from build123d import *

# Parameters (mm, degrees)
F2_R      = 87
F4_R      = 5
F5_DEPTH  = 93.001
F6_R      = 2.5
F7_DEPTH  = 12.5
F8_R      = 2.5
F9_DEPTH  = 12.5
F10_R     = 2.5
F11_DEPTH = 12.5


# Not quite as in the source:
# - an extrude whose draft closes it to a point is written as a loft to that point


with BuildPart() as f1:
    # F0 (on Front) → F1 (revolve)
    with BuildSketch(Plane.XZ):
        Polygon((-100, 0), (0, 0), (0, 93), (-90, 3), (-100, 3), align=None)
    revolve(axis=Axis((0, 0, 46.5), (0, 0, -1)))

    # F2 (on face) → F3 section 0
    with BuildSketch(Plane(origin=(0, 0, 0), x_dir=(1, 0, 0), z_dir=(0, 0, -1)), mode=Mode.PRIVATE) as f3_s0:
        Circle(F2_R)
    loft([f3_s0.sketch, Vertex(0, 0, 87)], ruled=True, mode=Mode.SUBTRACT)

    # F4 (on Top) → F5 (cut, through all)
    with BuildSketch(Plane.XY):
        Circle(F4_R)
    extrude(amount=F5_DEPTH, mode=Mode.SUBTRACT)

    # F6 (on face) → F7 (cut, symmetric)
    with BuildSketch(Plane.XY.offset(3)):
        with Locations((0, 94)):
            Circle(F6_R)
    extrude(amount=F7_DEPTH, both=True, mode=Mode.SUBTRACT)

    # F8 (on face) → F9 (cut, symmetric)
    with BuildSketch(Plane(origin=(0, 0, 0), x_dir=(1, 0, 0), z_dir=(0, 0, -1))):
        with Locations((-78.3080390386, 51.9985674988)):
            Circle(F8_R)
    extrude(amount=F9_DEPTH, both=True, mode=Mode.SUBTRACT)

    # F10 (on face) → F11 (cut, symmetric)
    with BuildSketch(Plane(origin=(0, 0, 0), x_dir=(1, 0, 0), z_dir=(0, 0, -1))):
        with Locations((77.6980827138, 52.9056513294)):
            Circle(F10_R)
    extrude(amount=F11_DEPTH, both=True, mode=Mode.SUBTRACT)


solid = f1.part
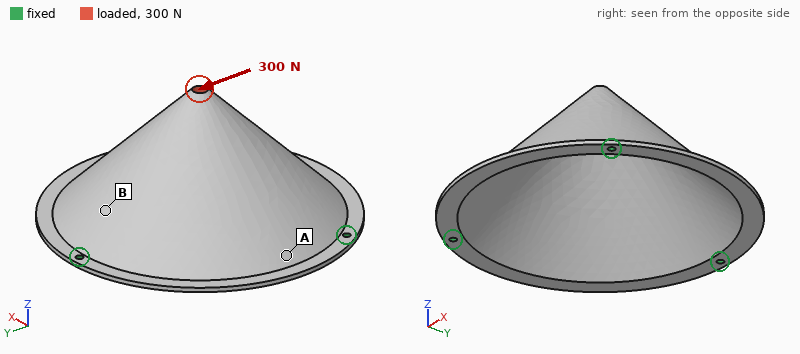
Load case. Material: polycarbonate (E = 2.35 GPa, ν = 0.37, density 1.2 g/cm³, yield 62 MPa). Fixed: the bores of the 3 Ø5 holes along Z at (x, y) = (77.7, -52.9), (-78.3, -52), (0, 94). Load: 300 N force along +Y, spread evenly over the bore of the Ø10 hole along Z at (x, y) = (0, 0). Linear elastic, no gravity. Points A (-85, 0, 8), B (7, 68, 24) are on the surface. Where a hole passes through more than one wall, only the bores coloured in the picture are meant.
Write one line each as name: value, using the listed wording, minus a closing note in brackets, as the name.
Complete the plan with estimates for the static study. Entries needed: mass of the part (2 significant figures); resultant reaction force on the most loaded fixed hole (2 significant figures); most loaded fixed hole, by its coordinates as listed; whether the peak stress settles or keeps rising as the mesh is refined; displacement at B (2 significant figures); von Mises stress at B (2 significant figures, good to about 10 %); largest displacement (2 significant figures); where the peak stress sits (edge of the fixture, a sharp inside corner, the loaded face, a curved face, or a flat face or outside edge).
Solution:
mass of the part: 200 g
resultant reaction force on the most loaded fixed hole: 260 N
most loaded fixed hole, by its coordinates as listed: (0, 94)
whether the peak stress settles or keeps rising as the mesh is refined: keeps rising
displacement at B: 0.10 mm
von Mises stress at B: 1.7 MPa
largest displacement: 0.19 mm
where the peak stress sits: edge of the fixture
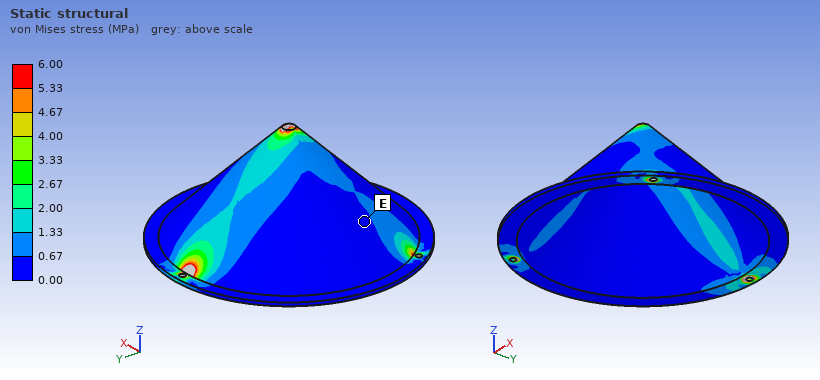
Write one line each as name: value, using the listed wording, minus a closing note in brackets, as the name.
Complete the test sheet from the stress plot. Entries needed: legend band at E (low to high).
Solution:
legend band at E: 0.00 to 0.67 MPa
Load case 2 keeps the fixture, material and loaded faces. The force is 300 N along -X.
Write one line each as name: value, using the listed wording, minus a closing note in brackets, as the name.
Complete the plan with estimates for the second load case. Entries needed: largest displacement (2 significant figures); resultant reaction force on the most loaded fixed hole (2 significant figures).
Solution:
largest displacement: 0.22 mm
resultant reaction force on the most loaded fixed hole: 250 N
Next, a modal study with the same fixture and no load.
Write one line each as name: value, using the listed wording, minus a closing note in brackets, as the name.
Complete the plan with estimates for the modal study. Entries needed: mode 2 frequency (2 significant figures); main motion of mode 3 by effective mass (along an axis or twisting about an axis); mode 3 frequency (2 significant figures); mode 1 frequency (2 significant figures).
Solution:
mode 2 frequency: 600 Hz
main motion of mode 3 by effective mass: twisting about Y
mode 3 frequency: 680 Hz
mode 1 frequency: 590 Hz
